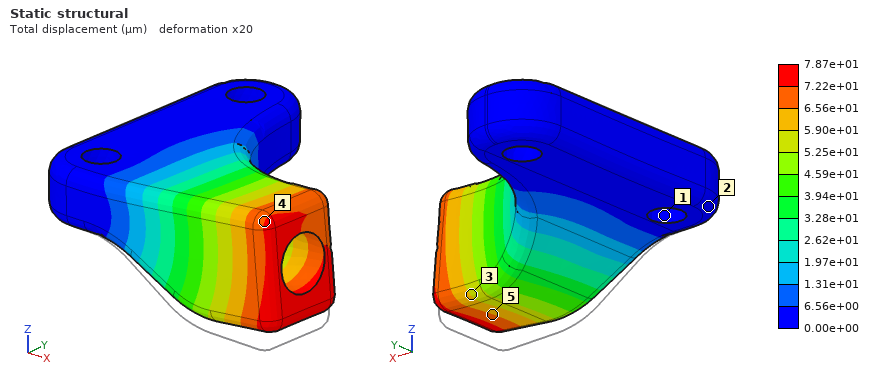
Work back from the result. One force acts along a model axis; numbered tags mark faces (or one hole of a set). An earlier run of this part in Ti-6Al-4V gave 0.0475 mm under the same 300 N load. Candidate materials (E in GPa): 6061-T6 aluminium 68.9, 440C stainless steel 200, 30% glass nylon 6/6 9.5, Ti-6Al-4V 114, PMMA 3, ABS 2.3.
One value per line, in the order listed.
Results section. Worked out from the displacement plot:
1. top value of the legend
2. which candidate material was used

7.87e+01 µm
6061-T6 aluminium
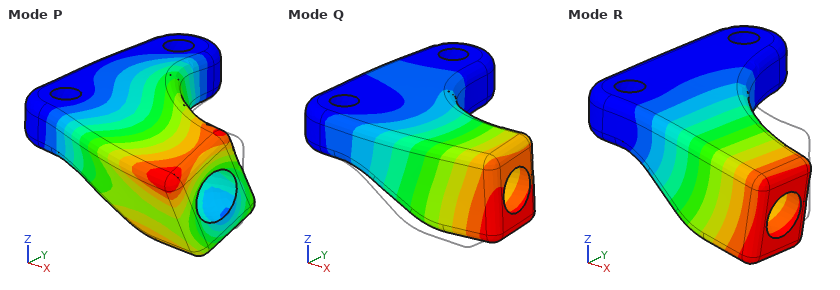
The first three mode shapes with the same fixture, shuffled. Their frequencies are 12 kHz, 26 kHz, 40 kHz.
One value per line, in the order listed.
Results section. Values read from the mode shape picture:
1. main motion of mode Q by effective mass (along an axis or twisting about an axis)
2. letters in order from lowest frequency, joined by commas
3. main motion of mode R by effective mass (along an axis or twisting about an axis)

along Y
R, Q, P
along Z
